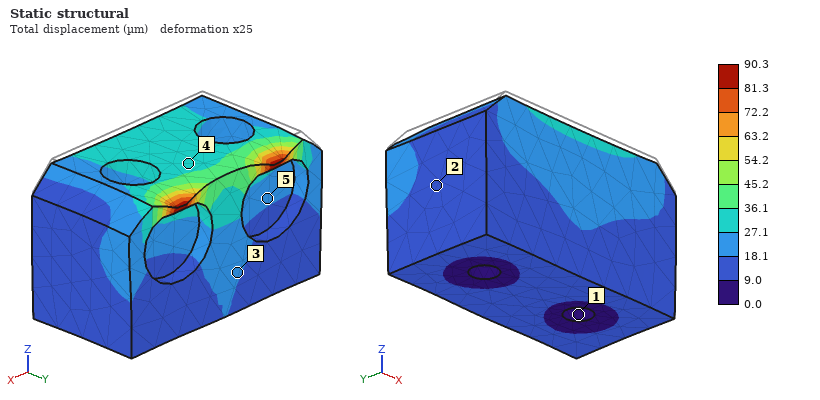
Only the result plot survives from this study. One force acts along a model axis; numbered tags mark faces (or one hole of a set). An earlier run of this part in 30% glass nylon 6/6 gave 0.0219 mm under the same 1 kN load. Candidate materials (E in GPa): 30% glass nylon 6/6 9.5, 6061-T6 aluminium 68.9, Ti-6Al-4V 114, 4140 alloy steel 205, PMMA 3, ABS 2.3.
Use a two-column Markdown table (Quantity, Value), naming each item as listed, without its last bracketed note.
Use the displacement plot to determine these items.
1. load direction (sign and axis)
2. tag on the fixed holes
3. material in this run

| Quantity | Value |
|---|---|
| load direction | -Z |
| tag on the fixed holes | 1 |
| material in this run | ABS |
